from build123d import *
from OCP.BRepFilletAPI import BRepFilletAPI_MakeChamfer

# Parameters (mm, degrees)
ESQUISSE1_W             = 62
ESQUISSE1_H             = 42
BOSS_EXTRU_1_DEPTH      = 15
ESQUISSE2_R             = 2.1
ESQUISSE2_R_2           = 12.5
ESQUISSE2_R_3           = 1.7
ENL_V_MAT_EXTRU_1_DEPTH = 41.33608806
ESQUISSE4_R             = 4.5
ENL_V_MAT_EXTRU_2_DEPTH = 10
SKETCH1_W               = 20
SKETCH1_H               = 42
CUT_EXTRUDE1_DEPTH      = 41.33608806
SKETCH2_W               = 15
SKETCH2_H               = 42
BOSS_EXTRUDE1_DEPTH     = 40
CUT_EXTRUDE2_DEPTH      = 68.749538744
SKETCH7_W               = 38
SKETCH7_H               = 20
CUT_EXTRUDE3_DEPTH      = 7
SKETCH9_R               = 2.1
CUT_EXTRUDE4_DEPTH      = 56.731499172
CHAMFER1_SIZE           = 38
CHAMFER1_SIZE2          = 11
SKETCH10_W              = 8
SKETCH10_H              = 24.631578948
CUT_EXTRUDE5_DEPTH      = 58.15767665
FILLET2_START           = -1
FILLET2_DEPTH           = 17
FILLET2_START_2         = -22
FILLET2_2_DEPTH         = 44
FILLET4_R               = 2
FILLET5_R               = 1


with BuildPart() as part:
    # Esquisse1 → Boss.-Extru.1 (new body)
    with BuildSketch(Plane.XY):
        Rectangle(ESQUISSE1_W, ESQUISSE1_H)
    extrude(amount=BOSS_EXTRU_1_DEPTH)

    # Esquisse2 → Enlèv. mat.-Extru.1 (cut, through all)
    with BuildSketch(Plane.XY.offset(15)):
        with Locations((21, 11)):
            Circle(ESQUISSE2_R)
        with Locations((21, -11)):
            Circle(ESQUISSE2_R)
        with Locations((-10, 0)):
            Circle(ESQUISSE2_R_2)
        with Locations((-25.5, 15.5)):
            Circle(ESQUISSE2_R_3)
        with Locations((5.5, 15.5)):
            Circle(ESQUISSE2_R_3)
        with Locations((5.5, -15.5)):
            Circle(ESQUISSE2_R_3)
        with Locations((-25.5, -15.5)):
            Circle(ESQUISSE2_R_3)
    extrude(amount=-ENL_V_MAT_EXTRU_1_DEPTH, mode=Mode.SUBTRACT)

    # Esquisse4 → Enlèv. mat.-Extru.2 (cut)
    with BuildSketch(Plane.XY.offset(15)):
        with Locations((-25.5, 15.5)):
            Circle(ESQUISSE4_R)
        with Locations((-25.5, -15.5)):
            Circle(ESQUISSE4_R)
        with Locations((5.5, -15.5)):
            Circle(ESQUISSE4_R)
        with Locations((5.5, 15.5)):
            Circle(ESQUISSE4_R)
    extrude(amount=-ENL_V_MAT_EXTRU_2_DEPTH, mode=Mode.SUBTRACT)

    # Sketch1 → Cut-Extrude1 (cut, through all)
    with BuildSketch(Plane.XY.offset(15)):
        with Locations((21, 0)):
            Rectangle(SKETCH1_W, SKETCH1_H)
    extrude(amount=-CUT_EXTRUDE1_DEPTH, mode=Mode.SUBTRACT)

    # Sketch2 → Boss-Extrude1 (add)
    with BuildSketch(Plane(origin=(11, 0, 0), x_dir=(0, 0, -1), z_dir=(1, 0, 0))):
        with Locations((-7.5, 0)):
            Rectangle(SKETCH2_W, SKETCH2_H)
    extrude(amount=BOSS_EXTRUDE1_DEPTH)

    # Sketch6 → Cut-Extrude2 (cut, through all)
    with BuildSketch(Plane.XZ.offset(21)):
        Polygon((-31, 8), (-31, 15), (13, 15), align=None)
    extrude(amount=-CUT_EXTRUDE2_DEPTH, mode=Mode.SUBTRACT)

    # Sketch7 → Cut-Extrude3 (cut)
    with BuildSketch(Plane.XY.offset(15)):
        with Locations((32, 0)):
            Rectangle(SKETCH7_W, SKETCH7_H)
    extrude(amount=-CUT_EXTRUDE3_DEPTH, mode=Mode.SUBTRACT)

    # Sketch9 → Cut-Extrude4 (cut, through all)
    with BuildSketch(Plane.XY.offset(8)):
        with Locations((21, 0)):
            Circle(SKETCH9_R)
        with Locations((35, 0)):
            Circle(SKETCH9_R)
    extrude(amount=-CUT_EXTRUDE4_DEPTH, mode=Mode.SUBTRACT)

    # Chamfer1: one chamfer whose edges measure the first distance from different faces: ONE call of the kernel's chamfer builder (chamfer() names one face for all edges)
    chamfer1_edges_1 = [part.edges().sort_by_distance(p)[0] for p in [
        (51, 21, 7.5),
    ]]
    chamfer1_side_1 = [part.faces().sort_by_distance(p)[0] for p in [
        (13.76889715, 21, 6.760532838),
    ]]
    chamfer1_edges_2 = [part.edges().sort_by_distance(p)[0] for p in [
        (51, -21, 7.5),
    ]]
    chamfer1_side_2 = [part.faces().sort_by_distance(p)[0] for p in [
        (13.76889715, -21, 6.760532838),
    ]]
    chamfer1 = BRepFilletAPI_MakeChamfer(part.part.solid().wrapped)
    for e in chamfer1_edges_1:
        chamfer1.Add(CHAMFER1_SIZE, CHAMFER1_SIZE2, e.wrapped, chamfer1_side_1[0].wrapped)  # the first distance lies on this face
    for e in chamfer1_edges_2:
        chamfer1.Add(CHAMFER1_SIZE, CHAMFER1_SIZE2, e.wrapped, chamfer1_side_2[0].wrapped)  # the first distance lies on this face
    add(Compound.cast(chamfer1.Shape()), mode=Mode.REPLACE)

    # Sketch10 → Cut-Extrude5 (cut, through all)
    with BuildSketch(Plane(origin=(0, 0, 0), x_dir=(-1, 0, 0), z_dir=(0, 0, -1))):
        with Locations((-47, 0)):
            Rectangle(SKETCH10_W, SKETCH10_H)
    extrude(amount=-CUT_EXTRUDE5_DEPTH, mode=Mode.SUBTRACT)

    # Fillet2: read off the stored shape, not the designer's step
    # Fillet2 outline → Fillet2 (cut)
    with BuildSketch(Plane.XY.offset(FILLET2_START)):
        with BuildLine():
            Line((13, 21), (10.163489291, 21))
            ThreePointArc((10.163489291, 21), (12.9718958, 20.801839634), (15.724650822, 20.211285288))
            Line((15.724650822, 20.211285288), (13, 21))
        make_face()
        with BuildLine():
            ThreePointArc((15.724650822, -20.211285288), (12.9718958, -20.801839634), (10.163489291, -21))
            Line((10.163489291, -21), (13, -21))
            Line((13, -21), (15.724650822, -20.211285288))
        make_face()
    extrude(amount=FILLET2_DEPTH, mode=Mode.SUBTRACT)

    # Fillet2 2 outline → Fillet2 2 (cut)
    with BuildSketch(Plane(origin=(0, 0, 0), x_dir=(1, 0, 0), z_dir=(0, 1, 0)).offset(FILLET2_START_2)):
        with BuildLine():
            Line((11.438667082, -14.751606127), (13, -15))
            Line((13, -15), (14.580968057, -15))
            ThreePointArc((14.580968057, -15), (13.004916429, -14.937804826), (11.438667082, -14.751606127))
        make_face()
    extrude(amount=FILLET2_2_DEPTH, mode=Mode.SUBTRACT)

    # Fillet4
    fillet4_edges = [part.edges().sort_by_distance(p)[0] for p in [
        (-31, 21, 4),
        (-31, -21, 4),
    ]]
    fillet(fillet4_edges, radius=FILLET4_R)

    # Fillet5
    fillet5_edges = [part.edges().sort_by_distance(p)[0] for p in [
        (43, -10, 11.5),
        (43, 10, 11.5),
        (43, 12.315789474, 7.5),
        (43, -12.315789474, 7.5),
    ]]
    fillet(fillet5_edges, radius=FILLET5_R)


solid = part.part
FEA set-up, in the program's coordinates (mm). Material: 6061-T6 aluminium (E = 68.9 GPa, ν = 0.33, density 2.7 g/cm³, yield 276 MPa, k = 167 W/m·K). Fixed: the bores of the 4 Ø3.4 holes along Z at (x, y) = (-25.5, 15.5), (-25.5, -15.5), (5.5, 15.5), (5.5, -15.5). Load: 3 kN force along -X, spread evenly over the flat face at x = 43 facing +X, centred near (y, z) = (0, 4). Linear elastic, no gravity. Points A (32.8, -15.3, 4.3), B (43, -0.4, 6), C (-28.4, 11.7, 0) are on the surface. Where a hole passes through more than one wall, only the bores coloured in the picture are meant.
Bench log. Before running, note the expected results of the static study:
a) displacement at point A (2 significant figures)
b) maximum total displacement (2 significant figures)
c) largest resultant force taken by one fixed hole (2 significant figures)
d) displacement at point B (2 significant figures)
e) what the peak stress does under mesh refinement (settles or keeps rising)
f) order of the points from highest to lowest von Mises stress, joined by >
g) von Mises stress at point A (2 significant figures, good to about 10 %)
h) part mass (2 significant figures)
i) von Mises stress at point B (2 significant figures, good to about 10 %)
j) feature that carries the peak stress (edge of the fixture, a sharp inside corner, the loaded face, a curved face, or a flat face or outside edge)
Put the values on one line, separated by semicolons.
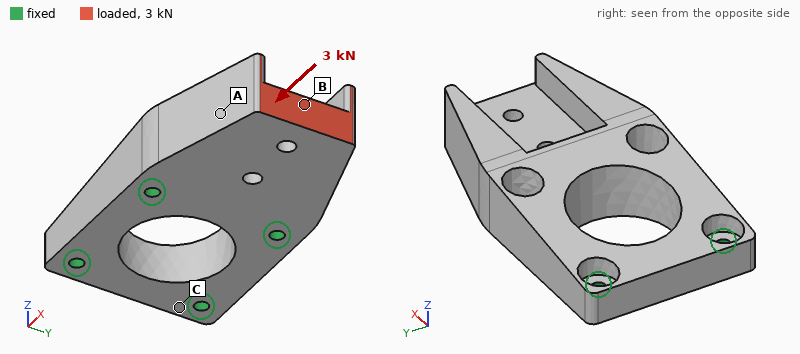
5.2 µm; 9.7 µm; 1.3 kN; 8.8 µm; keeps rising; B > A > C; 8.7 MPa; 66 g; 15 MPa; edge of the fixture
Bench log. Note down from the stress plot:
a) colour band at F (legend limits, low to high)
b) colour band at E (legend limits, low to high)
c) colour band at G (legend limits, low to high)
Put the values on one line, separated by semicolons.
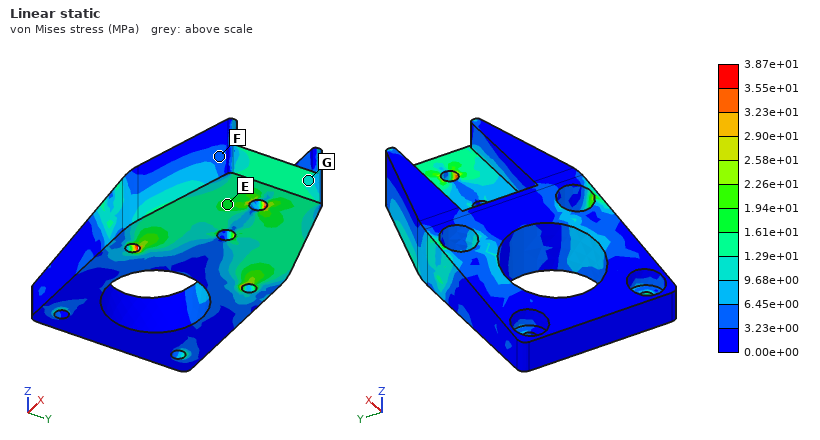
3.23e+00 to 6.45e+00 MPa; 1.61e+01 to 1.94e+01 MPa; 9.68e+00 to 1.29e+01 MPa
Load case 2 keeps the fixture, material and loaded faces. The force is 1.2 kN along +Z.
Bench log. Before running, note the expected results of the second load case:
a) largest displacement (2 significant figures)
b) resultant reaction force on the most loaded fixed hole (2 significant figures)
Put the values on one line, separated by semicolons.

0.14 mm; 1.4 kN
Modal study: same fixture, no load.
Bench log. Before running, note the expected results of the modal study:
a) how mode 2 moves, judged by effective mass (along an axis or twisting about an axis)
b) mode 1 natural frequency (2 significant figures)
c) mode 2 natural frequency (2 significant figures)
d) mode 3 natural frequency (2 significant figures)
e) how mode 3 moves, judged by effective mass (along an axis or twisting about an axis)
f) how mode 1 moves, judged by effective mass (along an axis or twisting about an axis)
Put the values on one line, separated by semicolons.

twisting about X; 5000 Hz; 12 kHz; 13 kHz; along Y; along Z
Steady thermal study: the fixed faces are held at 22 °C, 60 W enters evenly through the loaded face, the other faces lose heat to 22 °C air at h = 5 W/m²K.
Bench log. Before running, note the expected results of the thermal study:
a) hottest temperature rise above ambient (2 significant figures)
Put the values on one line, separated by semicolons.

52 K
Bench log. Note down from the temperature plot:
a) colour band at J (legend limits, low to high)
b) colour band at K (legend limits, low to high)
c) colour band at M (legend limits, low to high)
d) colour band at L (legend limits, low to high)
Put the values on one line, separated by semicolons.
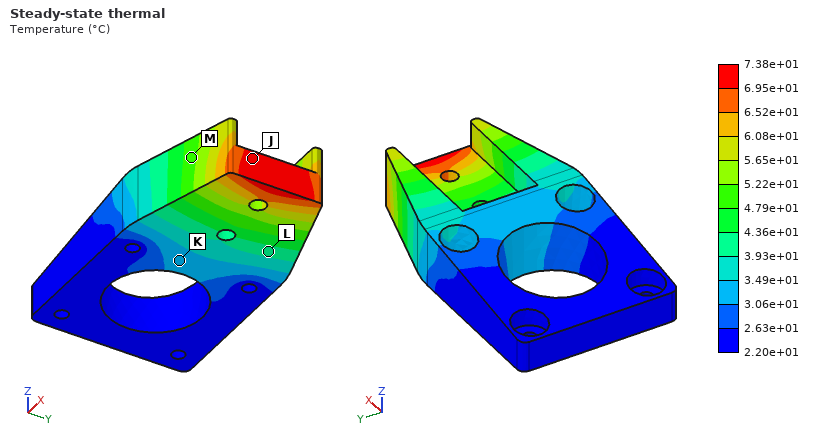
6.95e+01 to 7.38e+01 °C; 3.06e+01 to 3.49e+01 °C; 4.79e+01 to 5.22e+01 °C; 3.93e+01 to 4.36e+01 °C
